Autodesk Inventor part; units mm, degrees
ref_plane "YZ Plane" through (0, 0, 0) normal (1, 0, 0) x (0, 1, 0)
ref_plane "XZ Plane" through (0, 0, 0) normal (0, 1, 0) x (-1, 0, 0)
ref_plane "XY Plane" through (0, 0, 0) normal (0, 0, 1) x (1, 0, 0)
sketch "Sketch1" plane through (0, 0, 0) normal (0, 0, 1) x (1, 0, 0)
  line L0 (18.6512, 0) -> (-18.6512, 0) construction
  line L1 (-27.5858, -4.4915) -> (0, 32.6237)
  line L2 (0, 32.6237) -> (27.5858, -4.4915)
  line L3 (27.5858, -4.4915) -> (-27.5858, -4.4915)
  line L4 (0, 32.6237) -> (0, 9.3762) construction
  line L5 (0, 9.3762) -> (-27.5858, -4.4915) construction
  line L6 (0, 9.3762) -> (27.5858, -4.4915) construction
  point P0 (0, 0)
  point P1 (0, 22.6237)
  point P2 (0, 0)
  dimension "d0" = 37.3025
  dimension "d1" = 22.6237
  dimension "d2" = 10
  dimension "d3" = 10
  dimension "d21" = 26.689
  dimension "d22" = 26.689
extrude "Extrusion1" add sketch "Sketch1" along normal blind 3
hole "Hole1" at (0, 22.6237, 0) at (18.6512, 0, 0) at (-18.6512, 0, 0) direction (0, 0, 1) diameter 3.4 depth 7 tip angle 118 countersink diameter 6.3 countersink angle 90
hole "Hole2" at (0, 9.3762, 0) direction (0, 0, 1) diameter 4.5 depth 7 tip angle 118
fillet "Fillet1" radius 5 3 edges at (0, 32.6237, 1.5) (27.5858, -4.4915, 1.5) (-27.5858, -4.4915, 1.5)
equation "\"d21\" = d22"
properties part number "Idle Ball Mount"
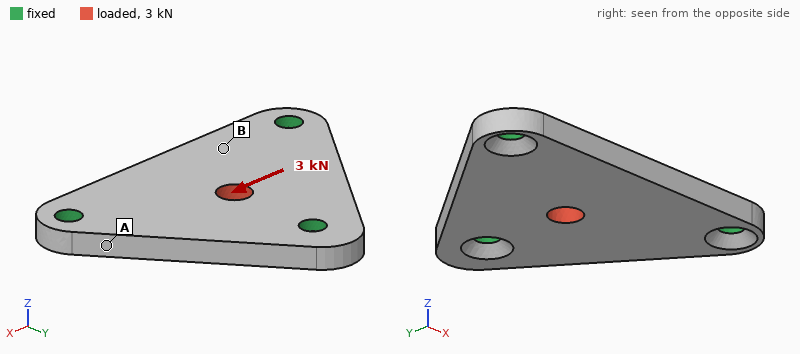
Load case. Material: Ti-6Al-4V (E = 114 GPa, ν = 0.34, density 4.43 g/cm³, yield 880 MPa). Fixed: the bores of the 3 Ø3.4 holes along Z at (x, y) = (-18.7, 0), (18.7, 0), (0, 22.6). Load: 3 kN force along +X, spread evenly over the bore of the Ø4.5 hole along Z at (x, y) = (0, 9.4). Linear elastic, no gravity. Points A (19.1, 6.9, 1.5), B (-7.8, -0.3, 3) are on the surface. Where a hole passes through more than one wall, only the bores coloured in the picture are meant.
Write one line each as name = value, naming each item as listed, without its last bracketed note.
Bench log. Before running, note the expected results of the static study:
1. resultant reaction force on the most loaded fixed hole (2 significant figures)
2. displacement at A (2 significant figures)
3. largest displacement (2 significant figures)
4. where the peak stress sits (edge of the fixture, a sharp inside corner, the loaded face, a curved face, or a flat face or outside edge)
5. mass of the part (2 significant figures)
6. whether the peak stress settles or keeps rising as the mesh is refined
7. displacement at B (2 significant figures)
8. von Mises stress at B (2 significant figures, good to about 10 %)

resultant reaction force on the most loaded fixed hole = 1.1 kN
displacement at A = 3.8 µm
largest displacement = 9.1 µm
where the peak stress sits = edge of the fixture
mass of the part = 12 g
whether the peak stress settles or keeps rising as the mesh is refined = keeps rising
displacement at B = 3.9 µm
von Mises stress at B = 30 MPa
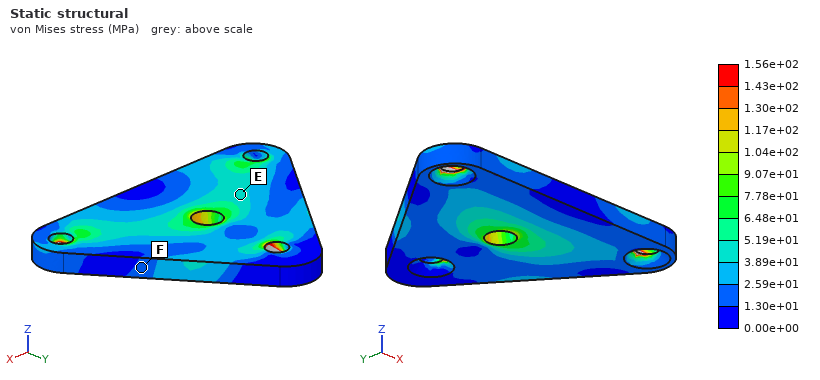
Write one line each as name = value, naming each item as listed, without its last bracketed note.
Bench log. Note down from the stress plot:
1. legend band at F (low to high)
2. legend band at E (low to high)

legend band at F = 1.30e+01 to 2.59e+01 MPa
legend band at E = 3.89e+01 to 5.19e+01 MPa
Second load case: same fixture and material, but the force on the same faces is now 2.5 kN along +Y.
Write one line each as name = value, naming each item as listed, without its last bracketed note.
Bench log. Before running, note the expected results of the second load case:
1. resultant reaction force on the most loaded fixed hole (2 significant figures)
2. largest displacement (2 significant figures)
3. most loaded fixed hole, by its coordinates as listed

resultant reaction force on the most loaded fixed hole = 1.6 kN
largest displacement = 9.7 µm
most loaded fixed hole, by its coordinates as listed = (0, 22.6)
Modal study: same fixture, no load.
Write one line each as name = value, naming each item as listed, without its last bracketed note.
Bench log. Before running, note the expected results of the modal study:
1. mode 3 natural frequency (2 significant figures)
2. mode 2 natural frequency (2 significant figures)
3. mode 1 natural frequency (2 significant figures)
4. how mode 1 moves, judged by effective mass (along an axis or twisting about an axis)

mode 3 natural frequency = 17 kHz
mode 2 natural frequency = 17 kHz
mode 1 natural frequency = 11 kHz
how mode 1 moves, judged by effective mass = along Z
